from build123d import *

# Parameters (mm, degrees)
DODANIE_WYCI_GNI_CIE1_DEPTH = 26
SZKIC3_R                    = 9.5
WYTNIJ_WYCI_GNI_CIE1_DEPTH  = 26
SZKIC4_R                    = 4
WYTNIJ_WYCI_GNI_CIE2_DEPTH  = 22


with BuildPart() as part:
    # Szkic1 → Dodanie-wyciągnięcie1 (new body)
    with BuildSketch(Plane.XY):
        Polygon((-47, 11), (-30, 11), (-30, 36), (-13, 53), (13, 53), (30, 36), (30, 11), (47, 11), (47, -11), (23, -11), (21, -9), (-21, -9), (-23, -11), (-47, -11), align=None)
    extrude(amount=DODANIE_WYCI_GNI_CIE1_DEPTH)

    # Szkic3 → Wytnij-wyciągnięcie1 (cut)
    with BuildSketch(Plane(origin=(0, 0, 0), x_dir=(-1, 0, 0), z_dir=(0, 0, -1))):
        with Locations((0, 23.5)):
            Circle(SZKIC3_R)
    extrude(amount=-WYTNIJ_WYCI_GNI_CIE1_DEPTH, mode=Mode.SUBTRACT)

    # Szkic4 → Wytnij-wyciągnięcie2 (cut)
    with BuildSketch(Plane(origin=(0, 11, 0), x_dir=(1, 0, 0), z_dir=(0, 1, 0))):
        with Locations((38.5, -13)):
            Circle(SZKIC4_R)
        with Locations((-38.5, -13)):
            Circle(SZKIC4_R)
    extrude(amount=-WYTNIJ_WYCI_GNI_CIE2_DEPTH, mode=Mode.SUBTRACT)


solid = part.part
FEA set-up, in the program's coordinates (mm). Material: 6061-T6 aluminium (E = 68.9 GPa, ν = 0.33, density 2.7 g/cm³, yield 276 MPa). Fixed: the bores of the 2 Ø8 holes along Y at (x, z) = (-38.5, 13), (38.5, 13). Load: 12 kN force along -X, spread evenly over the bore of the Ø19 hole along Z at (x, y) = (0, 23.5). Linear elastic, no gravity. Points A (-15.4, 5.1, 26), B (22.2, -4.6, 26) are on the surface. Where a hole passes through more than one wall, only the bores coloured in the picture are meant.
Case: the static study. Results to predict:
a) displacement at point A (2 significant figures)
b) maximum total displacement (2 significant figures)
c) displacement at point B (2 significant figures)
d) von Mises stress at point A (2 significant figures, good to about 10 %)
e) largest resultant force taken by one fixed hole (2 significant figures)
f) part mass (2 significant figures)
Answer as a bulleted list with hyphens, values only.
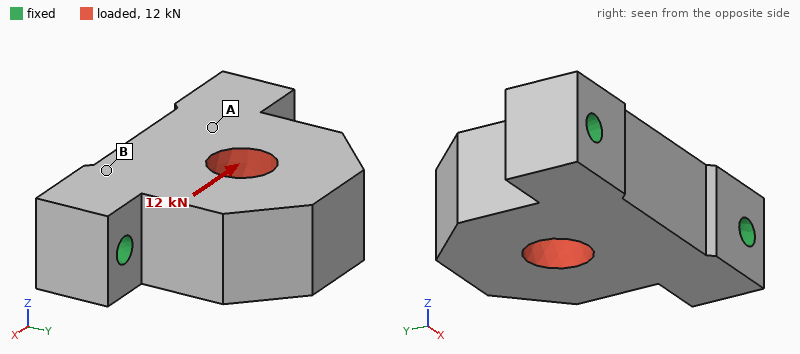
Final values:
- 3.5 µm
- 18 µm
- 2.9 µm
- 8.1 MPa
- 7.1 kN
- 270 g
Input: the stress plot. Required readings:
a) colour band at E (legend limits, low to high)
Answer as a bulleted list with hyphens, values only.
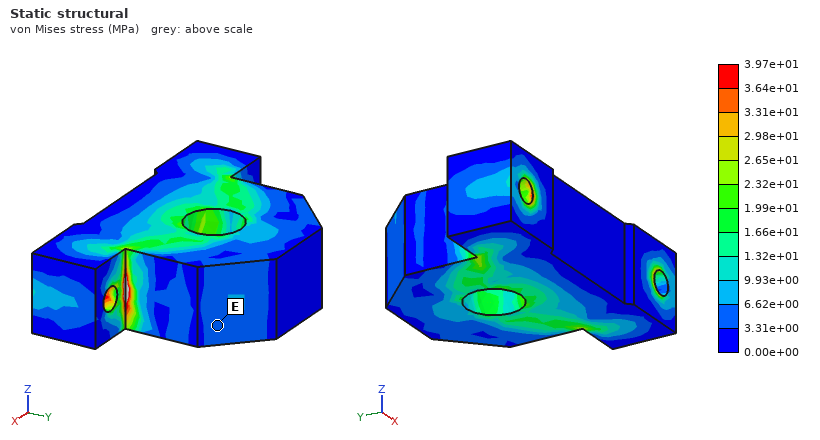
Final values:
- 3.31e+00 to 6.62e+00 MPa
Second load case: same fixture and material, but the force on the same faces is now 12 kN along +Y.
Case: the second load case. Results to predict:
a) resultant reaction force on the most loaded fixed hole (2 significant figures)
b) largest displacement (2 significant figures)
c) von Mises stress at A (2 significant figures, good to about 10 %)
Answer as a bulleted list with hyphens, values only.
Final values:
- 6.5 kN
- 14 µm
- 8.3 MPa
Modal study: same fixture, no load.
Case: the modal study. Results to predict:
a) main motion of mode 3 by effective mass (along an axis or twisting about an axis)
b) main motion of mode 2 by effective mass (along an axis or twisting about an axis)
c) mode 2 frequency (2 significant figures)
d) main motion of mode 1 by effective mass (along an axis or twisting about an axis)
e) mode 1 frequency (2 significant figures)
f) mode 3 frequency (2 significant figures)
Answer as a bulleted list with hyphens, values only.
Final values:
- along Y
- along X
- 10 kHz
- along Z
- 4100 Hz
- 11 kHz
